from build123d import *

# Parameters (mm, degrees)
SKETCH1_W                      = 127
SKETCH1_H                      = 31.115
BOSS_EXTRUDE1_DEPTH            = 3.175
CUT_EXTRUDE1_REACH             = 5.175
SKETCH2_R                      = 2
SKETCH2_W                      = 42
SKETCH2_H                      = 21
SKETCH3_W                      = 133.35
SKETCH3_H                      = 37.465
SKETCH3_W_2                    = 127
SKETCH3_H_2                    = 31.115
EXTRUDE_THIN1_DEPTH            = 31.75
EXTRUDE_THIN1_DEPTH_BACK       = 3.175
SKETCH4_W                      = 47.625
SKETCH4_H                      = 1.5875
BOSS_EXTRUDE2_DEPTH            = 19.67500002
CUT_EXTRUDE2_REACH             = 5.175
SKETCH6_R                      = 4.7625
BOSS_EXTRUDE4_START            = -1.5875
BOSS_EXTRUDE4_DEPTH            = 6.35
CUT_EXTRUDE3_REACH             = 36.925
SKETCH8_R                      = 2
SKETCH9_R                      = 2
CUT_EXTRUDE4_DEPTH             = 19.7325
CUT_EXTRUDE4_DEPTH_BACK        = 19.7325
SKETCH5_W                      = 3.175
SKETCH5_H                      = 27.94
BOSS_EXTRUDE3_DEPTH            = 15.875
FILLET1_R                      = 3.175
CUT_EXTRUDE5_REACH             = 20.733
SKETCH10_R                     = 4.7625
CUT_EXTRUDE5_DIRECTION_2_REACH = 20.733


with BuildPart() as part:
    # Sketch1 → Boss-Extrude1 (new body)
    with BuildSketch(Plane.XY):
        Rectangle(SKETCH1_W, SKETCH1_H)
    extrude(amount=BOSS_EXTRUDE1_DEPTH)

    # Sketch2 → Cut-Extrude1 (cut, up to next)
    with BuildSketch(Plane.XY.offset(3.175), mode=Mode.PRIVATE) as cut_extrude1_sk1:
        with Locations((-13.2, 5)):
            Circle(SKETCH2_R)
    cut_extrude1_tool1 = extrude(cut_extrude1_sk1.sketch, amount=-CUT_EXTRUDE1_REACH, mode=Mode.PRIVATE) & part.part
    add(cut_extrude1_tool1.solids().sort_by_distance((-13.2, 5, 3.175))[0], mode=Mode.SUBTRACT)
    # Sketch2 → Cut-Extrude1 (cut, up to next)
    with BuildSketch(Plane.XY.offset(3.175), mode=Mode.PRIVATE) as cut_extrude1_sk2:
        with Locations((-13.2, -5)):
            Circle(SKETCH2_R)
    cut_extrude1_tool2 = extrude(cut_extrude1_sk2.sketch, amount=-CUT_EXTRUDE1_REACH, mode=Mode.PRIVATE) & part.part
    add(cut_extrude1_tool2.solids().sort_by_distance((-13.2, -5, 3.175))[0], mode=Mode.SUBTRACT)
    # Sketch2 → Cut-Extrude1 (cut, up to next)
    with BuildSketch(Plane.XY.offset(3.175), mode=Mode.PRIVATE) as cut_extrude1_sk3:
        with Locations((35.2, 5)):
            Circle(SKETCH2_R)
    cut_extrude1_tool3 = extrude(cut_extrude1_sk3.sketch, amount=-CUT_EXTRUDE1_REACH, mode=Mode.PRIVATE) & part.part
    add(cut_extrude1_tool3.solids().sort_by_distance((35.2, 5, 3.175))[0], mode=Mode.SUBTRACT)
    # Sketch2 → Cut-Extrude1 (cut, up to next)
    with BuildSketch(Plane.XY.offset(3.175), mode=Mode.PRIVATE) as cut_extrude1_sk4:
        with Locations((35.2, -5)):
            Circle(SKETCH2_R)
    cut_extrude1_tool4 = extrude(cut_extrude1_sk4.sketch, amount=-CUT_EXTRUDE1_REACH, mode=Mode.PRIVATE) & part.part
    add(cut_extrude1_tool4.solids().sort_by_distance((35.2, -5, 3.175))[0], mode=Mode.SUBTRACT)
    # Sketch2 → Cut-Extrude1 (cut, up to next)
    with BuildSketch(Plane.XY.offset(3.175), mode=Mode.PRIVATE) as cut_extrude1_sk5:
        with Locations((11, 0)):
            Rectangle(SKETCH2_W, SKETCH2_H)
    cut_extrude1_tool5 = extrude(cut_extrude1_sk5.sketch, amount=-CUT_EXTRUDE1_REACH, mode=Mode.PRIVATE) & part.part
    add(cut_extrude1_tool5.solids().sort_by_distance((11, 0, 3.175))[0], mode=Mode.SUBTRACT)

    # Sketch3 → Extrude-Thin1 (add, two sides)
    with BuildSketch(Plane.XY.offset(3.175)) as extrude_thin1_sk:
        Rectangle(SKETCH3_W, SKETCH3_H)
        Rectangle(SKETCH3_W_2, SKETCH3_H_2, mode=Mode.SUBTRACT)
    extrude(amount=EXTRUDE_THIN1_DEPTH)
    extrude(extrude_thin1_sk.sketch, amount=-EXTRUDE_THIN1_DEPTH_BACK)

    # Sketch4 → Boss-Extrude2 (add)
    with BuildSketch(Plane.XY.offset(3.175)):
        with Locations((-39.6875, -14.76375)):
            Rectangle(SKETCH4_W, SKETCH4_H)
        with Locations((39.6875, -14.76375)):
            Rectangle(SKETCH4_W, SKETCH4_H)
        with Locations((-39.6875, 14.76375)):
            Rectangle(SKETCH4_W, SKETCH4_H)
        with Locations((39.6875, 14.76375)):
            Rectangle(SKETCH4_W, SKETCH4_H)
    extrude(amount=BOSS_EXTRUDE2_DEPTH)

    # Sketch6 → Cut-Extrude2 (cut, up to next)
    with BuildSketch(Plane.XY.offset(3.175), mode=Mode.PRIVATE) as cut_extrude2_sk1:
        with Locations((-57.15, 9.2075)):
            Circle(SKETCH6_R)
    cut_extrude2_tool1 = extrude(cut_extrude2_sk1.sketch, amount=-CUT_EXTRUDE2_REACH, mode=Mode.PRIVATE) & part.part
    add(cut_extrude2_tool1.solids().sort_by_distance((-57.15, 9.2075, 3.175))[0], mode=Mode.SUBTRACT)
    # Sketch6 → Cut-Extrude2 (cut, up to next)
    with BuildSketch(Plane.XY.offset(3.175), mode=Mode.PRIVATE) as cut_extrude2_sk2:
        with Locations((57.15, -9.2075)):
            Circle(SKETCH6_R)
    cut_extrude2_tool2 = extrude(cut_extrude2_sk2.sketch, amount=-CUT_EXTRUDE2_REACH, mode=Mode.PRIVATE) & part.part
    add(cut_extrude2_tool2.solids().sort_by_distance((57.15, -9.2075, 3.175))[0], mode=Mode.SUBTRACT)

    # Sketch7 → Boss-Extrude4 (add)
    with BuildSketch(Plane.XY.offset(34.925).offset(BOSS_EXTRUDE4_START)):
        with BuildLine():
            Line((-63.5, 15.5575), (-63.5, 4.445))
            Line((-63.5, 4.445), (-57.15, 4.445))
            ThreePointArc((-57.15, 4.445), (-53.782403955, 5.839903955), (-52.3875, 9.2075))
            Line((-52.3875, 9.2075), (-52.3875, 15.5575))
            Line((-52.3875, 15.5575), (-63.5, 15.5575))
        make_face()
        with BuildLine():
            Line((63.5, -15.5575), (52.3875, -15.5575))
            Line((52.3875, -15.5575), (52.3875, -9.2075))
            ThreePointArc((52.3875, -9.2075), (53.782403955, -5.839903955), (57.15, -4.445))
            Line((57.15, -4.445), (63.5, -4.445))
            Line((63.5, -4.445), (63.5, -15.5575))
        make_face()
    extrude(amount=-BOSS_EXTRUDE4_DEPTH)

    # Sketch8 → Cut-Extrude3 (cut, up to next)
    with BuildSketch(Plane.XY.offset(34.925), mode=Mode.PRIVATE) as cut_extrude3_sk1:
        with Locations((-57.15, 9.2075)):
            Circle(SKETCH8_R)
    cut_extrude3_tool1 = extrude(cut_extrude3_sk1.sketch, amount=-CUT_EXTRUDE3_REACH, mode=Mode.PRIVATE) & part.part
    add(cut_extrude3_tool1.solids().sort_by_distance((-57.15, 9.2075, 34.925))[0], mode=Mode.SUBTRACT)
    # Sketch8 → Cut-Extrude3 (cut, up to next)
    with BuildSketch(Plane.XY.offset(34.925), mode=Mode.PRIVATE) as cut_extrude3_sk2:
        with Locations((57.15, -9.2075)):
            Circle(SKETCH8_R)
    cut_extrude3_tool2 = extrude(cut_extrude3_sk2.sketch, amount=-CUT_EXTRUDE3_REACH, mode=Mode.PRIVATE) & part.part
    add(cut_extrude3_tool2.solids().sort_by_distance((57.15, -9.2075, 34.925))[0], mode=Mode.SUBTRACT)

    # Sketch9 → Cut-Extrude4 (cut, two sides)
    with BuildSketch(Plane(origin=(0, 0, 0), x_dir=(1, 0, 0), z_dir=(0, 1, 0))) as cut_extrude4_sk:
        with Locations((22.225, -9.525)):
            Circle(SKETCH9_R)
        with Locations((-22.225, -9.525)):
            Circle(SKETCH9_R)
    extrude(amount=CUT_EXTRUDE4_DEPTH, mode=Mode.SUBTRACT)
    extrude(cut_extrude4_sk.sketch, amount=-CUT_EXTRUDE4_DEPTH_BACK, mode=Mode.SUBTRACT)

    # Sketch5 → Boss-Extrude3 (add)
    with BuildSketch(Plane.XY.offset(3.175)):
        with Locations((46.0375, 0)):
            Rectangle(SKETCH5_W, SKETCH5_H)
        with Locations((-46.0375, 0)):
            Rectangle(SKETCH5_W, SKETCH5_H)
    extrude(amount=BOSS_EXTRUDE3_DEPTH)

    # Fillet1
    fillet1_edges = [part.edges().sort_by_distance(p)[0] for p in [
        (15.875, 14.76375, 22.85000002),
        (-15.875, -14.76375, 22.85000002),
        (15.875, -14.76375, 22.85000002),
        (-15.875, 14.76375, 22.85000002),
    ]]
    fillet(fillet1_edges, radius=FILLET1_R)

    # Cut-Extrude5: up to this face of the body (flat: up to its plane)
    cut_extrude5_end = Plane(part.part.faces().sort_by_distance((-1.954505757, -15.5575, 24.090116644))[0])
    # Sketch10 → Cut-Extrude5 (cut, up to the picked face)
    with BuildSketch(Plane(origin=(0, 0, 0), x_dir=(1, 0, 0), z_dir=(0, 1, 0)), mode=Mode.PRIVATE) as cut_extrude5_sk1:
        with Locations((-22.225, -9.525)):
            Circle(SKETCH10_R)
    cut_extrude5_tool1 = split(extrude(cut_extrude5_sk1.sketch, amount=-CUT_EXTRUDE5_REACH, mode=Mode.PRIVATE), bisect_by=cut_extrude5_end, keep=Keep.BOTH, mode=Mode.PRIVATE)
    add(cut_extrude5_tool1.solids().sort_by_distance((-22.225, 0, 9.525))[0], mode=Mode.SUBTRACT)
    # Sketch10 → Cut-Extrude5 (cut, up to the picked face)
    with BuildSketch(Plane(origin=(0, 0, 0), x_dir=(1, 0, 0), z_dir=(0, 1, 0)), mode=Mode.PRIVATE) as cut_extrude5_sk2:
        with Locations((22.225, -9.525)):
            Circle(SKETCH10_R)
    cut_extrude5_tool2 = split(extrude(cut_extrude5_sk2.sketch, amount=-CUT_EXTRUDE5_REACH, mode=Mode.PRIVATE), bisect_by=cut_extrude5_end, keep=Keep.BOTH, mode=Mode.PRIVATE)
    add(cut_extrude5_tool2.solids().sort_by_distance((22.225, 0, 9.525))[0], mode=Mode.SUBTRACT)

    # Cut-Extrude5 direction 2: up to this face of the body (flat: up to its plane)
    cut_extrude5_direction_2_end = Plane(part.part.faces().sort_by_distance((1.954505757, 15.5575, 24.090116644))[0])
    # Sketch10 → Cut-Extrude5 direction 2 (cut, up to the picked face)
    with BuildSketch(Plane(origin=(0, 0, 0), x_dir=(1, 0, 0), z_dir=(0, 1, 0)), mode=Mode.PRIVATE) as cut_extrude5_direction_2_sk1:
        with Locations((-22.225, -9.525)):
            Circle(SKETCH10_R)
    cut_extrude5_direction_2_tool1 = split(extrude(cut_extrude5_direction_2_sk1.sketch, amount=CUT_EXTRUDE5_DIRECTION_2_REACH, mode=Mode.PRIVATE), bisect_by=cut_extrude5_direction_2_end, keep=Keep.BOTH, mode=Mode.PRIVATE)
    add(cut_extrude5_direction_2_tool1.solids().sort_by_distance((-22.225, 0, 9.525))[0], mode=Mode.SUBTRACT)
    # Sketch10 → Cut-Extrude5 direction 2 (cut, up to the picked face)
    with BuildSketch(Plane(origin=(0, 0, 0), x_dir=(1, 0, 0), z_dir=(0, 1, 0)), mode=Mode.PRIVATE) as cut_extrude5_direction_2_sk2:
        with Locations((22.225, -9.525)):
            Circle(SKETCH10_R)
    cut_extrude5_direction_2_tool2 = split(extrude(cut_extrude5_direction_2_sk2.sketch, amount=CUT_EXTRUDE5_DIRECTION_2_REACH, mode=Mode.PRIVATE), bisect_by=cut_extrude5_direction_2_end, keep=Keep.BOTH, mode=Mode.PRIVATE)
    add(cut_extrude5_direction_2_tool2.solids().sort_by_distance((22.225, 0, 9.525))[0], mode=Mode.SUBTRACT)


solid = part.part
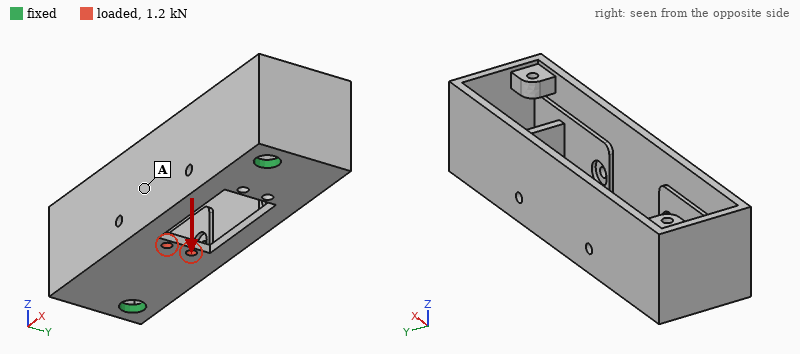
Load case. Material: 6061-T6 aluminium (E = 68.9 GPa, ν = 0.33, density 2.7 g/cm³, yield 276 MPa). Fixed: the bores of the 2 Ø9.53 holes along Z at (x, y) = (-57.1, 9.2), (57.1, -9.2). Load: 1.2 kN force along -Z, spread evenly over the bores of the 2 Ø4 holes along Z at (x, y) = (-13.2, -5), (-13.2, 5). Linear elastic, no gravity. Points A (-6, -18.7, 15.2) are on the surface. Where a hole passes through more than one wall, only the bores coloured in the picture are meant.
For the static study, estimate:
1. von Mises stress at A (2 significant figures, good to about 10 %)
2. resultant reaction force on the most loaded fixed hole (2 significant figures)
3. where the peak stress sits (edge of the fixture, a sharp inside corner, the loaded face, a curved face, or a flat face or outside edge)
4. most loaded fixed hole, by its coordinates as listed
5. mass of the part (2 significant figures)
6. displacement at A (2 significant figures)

19 MPa
860 N
the loaded face
(-57.1, 9.2)
150 g
0.041 mm
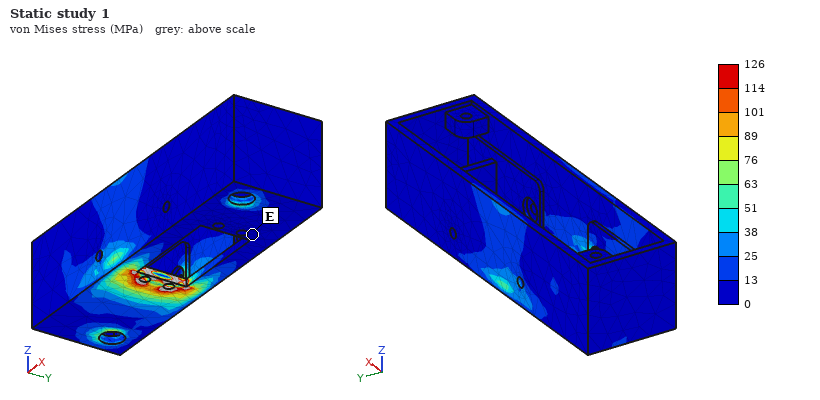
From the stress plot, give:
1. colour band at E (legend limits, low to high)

0 to 13 MPa
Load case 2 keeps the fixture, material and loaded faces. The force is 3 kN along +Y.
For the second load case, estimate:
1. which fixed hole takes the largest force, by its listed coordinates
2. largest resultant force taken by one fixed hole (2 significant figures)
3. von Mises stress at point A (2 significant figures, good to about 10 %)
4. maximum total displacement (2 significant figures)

(-57.1, 9.2)
2.9 kN
37 MPa
0.12 mm
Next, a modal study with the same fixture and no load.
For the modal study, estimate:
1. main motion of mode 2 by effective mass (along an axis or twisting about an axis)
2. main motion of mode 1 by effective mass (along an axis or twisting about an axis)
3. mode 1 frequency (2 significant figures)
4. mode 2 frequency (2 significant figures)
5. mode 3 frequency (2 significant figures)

along Z
along Y
1900 Hz
2600 Hz
2900 Hz
